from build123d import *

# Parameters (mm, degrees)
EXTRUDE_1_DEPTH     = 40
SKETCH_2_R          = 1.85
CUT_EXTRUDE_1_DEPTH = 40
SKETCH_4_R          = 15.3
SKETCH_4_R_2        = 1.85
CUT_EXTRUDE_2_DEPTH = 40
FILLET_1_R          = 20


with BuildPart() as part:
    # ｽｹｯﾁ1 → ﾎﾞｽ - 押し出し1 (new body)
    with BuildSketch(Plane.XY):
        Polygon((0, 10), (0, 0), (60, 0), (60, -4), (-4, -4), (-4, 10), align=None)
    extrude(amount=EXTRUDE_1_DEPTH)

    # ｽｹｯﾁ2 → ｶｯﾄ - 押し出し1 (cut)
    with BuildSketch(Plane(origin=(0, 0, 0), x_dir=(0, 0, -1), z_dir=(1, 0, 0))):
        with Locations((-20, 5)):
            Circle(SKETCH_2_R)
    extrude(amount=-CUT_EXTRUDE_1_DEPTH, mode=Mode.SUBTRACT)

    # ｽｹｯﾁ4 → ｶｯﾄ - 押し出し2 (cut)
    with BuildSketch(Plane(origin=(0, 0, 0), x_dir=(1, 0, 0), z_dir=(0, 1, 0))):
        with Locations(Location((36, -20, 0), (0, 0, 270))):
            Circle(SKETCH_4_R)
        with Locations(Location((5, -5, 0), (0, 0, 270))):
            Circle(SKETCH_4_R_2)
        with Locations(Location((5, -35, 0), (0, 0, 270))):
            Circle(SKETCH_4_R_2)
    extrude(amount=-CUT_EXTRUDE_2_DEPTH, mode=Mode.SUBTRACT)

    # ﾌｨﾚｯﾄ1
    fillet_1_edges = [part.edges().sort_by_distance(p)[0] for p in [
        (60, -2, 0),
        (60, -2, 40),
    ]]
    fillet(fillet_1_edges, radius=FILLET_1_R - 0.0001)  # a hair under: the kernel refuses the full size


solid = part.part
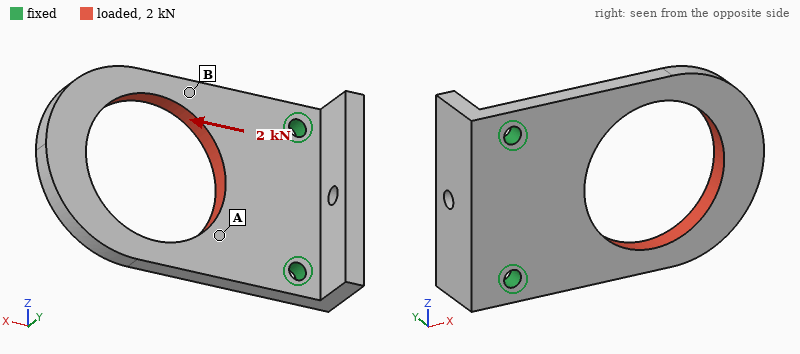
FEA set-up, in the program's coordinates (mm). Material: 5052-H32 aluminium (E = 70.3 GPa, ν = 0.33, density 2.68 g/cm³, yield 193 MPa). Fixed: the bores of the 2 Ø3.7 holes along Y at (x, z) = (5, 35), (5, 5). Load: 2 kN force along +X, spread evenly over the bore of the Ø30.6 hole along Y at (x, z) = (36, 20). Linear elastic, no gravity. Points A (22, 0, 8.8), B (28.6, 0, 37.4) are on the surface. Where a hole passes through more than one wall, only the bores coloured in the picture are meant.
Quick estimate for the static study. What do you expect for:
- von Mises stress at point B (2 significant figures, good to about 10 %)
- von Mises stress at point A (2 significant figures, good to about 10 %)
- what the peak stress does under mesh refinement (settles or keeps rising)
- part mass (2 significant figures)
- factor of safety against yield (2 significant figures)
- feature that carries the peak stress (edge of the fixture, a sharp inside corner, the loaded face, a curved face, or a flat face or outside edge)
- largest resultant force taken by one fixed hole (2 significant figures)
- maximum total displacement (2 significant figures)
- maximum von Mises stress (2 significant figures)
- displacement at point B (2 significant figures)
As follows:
31 MPa
11 MPa
settles
22 g
2.7
the loaded face
1.0 kN
32 µm
71 MPa
13 µm
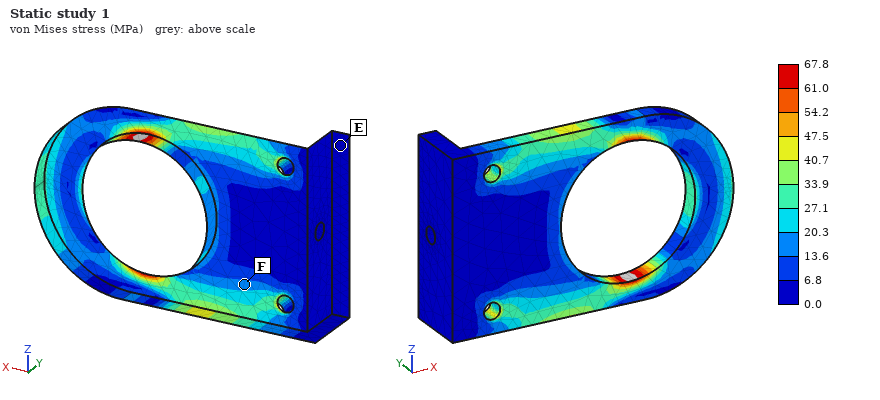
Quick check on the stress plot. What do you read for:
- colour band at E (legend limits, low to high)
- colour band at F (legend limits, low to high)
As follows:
0.0 to 6.8 MPa
13.6 to 20.3 MPa
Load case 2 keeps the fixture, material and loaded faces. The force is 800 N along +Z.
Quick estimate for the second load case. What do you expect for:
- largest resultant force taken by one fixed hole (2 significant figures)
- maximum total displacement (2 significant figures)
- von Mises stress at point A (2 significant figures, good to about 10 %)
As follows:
880 N
90 µm
25 MPa
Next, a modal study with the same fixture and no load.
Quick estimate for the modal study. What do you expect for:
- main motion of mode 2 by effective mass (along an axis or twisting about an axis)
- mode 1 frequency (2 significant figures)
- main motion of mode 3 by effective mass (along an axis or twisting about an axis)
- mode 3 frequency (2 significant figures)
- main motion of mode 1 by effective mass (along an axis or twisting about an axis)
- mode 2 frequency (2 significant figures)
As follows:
twisting about X
1200 Hz
along Z
5400 Hz
along Y
3500 Hz
